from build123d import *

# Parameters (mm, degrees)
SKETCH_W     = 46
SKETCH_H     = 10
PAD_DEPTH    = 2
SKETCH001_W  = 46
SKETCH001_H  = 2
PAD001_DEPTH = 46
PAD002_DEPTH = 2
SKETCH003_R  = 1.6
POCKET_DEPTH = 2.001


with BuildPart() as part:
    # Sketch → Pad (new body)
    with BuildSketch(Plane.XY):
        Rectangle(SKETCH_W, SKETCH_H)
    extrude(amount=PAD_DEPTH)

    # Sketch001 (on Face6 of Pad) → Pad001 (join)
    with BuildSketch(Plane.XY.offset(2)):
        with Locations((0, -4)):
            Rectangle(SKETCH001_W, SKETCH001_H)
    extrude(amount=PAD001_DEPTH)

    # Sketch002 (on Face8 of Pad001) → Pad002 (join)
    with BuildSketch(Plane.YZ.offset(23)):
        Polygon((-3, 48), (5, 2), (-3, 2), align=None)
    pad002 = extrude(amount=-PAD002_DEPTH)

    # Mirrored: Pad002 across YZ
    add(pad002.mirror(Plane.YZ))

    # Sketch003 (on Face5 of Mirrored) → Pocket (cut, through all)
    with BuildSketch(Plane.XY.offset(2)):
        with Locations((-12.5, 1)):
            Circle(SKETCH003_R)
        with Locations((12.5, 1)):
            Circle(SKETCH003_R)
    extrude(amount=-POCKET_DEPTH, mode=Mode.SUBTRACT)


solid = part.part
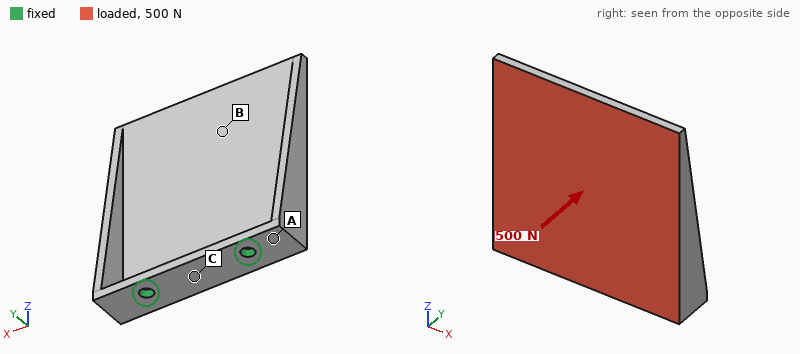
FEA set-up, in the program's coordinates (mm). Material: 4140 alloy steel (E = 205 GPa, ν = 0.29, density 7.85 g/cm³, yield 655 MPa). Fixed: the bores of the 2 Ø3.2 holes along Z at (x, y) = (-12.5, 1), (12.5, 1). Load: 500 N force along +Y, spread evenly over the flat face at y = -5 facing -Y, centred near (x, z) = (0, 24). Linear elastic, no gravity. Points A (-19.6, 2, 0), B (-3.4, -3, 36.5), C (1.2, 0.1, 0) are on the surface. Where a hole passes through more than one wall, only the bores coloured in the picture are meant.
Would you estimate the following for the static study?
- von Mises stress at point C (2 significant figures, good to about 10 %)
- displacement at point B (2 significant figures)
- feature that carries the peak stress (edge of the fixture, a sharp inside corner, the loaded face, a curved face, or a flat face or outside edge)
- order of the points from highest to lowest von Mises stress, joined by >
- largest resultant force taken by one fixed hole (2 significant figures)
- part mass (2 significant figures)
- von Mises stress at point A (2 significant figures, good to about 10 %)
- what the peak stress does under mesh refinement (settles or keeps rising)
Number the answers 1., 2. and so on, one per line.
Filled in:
1. 87 MPa
2. 0.43 mm
3. edge of the fixture
4. A > C > B
5. 270 N
6. 46 g
7. 290 MPa
8. keeps rising
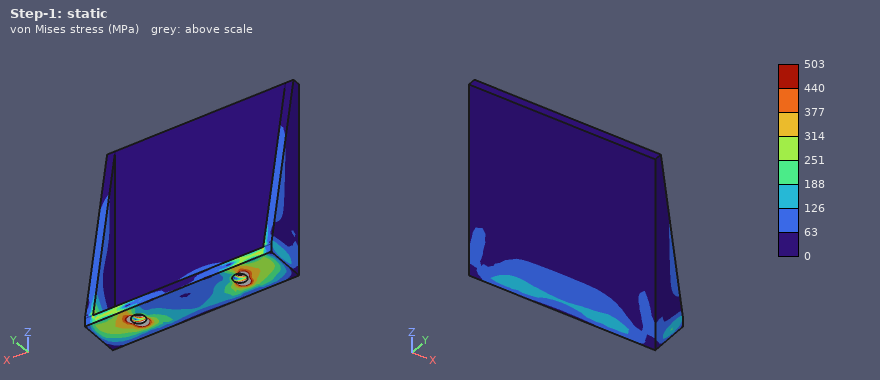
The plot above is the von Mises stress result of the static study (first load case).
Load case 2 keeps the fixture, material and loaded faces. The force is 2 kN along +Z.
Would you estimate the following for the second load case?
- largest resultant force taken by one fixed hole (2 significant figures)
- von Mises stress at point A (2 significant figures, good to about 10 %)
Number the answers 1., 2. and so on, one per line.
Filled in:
1. 1.0 kN
2. 130 MPa
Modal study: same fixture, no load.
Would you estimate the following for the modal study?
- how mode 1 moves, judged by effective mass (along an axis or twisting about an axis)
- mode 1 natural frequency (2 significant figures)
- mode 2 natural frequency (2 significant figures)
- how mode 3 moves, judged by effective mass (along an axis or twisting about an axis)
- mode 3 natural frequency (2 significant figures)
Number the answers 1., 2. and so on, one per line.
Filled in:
1. along Y
2. 950 Hz
3. 2000 Hz
4. along X
5. 4500 Hz
